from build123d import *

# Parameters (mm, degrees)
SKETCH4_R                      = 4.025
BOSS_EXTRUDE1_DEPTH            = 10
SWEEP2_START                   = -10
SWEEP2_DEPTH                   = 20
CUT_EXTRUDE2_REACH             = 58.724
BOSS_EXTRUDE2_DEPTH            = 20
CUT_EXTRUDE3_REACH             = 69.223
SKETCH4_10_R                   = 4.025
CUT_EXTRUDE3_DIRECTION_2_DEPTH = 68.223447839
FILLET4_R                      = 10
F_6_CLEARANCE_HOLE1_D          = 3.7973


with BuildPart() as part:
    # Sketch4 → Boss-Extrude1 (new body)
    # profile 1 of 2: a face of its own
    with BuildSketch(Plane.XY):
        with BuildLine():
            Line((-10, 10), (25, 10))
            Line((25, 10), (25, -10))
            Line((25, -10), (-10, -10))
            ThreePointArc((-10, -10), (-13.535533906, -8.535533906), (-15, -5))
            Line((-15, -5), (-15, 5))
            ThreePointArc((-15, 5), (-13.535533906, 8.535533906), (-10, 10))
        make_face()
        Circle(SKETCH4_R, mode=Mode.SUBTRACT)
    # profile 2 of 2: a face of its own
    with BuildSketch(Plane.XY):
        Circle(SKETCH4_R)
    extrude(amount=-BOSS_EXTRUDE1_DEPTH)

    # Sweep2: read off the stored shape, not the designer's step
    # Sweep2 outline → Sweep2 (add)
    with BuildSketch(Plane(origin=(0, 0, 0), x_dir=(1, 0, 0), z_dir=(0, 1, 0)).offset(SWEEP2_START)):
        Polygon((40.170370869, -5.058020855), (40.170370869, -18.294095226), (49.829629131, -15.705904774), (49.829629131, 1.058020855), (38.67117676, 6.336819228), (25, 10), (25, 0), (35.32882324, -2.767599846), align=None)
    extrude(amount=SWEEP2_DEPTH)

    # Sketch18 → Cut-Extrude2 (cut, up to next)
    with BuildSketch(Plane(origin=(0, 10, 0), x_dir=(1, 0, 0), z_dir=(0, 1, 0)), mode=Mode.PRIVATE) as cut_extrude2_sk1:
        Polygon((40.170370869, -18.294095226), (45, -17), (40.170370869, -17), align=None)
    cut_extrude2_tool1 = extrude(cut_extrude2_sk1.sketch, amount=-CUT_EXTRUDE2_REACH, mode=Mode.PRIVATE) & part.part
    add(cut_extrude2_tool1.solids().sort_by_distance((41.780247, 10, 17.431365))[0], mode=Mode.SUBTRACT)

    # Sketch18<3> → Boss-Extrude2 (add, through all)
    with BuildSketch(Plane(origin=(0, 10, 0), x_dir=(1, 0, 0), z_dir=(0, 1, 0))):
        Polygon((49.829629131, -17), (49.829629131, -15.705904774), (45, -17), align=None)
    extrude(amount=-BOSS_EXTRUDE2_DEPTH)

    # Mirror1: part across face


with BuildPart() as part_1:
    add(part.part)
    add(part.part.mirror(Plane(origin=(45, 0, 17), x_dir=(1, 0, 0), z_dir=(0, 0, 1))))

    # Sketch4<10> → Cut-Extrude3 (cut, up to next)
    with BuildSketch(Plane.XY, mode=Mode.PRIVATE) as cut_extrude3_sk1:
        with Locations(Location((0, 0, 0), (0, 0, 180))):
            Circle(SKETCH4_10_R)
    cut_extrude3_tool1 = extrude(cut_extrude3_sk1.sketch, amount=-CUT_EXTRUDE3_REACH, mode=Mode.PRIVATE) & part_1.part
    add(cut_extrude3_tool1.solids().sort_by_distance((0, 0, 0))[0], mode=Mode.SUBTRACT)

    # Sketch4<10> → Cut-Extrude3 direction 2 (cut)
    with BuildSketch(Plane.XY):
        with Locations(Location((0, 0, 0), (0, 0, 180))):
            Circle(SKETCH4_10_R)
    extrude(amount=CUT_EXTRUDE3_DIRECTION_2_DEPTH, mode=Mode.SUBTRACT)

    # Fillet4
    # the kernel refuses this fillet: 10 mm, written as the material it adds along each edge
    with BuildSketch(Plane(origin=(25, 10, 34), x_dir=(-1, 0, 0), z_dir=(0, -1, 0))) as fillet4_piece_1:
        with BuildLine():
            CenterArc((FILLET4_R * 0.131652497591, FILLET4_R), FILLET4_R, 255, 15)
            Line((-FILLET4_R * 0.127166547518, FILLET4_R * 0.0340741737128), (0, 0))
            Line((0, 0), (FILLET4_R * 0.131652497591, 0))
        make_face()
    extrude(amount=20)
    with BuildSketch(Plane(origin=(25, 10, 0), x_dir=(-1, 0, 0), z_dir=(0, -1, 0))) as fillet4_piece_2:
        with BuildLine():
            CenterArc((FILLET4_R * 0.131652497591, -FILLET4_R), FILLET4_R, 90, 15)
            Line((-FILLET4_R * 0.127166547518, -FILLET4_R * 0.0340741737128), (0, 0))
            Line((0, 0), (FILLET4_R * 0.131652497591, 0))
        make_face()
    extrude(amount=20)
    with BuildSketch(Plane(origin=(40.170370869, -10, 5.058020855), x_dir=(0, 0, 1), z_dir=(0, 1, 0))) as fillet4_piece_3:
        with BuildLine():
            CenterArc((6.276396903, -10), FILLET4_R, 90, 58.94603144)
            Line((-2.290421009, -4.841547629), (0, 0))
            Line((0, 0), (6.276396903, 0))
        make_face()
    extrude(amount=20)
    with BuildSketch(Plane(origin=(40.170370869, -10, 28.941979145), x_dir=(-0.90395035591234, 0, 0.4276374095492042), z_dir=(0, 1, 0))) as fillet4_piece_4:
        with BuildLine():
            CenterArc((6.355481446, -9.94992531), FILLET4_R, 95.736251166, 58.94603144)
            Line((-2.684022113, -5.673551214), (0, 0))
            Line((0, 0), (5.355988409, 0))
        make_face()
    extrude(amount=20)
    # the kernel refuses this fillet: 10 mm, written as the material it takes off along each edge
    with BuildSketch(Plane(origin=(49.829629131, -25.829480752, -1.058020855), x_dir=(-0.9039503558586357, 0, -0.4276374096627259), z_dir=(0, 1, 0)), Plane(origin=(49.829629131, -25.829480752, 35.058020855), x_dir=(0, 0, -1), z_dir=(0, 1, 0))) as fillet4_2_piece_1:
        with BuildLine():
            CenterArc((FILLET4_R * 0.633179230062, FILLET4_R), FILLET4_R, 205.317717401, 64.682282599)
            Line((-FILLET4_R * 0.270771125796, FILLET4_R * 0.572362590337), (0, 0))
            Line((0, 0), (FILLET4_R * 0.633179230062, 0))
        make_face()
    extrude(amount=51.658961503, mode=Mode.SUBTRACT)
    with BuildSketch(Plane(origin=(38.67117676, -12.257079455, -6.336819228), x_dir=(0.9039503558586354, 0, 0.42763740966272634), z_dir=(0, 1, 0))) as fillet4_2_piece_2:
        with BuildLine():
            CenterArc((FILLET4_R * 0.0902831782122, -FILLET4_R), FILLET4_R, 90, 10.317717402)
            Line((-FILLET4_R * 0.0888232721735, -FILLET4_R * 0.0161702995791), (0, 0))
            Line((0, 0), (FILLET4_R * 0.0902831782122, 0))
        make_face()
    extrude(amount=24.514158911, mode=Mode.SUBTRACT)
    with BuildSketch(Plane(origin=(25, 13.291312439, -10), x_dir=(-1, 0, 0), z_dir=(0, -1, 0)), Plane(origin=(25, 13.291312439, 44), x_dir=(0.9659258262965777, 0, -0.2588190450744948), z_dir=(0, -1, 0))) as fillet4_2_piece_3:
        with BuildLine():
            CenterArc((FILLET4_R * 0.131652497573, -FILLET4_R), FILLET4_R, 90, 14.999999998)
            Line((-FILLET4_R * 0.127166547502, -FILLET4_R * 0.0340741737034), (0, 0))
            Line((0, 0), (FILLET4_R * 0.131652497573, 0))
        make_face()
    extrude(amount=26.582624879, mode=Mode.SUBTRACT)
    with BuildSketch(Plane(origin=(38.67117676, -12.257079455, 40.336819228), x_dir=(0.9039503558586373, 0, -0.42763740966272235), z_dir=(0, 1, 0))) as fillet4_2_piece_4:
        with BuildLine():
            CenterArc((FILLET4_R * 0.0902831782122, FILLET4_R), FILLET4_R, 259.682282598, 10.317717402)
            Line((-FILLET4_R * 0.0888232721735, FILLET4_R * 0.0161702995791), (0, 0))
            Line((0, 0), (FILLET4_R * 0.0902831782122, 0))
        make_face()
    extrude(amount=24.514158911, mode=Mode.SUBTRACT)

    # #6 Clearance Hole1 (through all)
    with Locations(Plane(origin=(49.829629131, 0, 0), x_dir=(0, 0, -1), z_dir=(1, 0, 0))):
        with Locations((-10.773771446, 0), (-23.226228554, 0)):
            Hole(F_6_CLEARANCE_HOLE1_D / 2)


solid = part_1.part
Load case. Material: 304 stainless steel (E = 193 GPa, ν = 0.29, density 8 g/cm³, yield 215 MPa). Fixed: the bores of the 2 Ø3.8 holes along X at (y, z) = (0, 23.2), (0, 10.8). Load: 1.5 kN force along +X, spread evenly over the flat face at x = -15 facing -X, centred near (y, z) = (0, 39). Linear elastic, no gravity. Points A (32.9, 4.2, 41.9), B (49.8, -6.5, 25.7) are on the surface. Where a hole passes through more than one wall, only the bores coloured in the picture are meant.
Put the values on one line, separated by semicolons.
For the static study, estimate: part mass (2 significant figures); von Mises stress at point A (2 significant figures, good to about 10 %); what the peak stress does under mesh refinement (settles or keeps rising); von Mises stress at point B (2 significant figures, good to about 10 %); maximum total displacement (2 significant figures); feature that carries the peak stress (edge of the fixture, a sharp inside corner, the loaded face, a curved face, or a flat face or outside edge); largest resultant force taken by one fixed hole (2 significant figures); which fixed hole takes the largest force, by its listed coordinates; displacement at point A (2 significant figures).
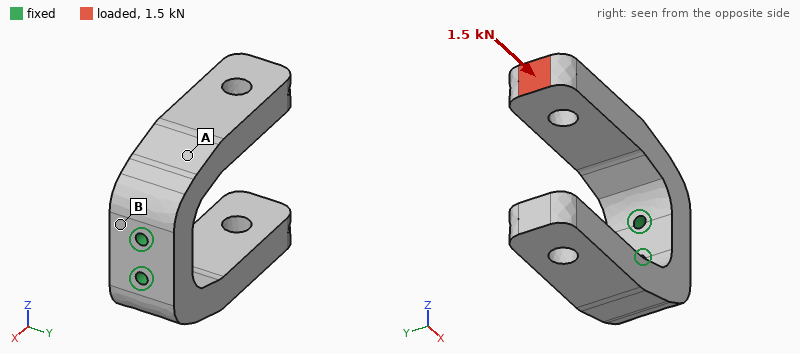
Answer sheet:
230 g; 16 MPa; keeps rising; 37 MPa; 49 µm; edge of the fixture; 1.9 kN; (0, 23.2); 14 µm
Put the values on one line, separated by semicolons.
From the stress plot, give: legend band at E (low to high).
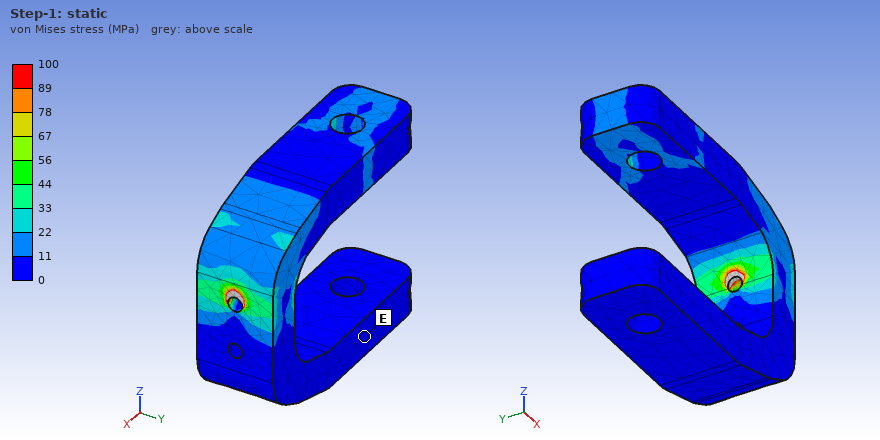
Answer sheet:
0 to 11 MPa
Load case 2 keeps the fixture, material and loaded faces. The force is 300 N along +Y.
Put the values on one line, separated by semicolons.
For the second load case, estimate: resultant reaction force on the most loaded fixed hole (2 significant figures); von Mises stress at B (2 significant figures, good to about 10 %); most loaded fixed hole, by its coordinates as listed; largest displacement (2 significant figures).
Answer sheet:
540 N; 27 MPa; (0, 23.2); 49 µm
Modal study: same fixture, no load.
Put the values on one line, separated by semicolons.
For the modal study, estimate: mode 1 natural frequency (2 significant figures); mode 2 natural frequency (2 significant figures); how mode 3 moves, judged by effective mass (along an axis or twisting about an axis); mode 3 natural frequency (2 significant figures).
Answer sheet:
1800 Hz; 1800 Hz; along Y; 2400 Hz
